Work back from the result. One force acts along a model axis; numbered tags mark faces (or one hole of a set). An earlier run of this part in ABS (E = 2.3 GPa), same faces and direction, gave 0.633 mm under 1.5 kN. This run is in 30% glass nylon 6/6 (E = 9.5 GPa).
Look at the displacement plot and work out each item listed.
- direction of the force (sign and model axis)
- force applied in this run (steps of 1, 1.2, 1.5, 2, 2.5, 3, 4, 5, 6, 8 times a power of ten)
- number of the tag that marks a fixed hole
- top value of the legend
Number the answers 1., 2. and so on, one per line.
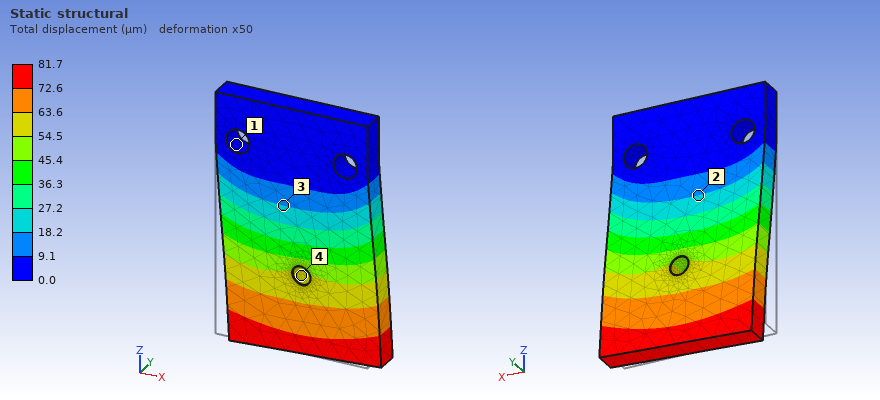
1. +X
2. 800 N
3. 1
4. 81.7 µm
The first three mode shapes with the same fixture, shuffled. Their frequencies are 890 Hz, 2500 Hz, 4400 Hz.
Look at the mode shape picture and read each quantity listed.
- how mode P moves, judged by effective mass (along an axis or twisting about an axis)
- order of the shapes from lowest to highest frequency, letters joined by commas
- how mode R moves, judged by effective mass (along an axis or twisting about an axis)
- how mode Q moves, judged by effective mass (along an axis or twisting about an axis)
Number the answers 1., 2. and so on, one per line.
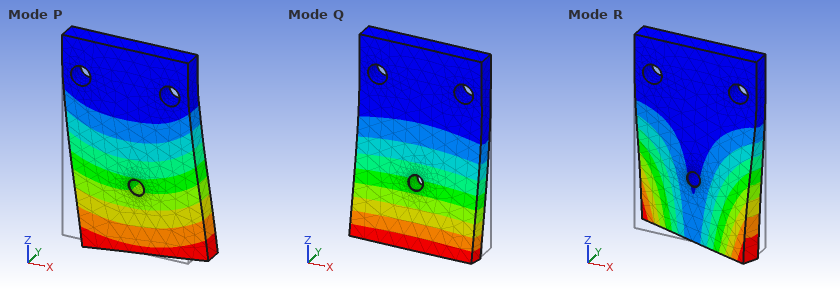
1. along X
2. Q, R, P
3. twisting about Z
4. along Y
